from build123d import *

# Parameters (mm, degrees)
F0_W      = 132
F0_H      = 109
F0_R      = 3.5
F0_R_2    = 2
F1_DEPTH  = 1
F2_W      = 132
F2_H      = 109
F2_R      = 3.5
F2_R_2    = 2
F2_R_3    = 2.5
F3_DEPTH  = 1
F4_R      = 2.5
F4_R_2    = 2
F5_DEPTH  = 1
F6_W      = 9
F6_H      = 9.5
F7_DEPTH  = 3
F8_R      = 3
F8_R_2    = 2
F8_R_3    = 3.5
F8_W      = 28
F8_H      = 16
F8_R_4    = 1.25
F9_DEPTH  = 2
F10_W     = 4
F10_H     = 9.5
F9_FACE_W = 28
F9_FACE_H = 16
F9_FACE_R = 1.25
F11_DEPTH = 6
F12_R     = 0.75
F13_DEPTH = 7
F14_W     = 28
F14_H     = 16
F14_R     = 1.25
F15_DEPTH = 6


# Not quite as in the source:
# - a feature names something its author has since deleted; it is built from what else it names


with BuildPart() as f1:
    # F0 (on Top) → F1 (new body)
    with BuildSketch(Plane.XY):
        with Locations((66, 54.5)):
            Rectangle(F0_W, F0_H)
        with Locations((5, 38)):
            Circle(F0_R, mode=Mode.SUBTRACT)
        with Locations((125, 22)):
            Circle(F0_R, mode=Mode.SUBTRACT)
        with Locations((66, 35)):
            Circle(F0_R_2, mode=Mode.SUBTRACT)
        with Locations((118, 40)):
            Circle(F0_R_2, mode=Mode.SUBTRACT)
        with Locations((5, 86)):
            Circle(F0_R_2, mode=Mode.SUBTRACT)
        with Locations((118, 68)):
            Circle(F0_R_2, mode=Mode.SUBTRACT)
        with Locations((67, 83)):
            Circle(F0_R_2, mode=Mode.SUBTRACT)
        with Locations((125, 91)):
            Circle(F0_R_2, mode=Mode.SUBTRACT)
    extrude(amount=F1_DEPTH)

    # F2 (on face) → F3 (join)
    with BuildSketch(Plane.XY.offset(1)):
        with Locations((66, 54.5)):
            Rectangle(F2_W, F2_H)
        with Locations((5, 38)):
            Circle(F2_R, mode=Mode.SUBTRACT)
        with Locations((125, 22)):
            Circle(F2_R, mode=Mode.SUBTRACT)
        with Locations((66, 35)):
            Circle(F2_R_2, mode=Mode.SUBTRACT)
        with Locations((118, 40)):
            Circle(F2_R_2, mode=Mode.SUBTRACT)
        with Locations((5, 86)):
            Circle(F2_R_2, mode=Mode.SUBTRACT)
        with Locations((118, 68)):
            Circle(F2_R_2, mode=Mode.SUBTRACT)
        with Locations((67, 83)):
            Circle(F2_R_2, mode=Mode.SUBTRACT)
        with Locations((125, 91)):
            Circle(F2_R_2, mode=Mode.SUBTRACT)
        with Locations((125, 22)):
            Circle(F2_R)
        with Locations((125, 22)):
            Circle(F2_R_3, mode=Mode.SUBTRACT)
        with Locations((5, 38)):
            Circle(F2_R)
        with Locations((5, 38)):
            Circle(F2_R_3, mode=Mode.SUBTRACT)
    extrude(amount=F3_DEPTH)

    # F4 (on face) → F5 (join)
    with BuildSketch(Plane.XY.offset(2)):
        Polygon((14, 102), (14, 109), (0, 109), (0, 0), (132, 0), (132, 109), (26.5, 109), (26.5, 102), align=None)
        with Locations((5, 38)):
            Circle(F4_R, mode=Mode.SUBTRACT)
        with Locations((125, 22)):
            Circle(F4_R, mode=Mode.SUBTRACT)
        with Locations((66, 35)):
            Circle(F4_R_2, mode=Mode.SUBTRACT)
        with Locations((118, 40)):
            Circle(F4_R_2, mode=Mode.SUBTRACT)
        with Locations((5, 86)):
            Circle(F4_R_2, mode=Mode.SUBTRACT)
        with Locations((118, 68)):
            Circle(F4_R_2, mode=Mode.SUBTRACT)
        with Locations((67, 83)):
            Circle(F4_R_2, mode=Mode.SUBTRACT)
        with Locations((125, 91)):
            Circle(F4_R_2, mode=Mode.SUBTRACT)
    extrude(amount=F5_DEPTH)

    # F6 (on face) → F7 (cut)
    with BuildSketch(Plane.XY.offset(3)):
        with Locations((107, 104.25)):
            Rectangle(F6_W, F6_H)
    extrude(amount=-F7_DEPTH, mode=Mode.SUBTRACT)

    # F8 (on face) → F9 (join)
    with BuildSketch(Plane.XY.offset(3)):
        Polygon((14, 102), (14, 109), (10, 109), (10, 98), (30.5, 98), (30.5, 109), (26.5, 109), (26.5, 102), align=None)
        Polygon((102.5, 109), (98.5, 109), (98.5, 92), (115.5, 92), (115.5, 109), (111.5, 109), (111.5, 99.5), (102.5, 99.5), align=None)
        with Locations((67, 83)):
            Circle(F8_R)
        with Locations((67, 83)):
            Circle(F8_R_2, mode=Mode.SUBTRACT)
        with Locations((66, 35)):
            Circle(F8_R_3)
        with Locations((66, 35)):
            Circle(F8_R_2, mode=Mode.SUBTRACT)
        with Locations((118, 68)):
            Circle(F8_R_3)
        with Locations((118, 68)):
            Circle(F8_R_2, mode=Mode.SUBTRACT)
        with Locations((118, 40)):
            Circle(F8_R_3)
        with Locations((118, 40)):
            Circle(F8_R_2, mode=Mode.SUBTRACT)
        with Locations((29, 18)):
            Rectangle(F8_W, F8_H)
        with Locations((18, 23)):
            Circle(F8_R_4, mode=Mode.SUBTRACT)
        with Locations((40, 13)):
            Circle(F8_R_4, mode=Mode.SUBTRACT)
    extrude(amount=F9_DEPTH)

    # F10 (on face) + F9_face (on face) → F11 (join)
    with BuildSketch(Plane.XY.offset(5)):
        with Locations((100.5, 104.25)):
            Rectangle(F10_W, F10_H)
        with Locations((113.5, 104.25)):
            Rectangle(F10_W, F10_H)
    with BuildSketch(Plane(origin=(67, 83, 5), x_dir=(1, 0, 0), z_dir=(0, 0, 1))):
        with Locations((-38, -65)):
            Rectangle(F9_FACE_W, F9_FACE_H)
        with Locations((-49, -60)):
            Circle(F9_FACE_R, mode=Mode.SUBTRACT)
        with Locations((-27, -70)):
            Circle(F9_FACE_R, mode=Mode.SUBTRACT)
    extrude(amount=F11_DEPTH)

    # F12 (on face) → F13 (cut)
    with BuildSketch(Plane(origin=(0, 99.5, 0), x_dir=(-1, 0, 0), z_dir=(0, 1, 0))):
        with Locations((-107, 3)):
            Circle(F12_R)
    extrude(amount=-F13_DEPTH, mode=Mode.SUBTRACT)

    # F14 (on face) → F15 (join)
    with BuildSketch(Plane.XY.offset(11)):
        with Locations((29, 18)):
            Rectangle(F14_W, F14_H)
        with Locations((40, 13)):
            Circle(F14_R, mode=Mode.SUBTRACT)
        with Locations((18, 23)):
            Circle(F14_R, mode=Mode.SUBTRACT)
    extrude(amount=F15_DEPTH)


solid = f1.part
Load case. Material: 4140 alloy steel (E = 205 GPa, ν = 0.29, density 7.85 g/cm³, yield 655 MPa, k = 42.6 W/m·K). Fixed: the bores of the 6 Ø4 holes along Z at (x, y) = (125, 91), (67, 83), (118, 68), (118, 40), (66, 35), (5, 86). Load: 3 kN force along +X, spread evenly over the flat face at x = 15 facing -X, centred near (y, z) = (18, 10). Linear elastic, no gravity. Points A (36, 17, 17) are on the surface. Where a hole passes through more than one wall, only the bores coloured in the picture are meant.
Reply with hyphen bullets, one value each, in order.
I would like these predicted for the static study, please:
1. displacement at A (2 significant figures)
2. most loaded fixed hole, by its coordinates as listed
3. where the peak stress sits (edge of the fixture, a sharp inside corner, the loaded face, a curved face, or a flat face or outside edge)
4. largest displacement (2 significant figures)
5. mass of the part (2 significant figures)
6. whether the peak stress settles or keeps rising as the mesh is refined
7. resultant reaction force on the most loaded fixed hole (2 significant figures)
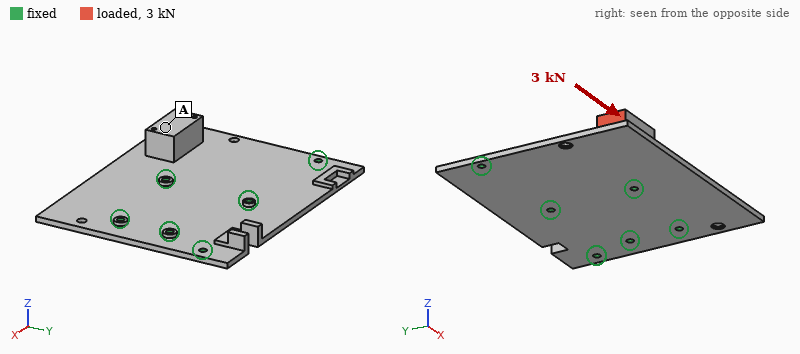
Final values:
- 0.34 mm
- (66, 35)
- edge of the fixture
- 0.84 mm
- 390 g
- keeps rising
- 2.1 kN
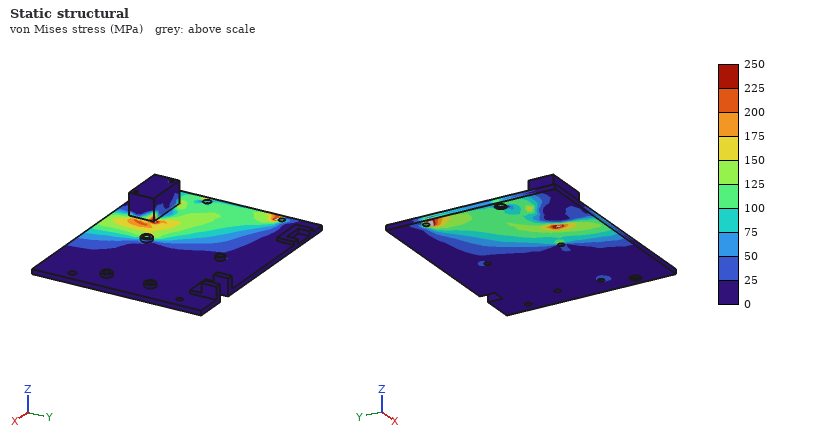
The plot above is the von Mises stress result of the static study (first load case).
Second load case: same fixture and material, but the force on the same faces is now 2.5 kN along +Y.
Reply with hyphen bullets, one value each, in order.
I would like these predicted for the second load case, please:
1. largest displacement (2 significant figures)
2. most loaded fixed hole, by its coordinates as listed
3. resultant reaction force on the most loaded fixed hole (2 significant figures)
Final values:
- 0.61 mm
- (5, 86)
- 1.3 kN
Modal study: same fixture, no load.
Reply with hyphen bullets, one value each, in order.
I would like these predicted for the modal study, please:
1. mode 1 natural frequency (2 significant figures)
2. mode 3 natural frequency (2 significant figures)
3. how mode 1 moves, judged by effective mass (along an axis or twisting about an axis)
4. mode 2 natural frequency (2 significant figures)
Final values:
- 620 Hz
- 2000 Hz
- along Z
- 1600 Hz
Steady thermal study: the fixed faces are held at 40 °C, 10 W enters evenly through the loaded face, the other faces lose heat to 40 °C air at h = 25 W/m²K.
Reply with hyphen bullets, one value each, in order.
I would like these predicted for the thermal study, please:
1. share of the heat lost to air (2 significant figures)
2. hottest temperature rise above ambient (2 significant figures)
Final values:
- 56 %
- 42 K
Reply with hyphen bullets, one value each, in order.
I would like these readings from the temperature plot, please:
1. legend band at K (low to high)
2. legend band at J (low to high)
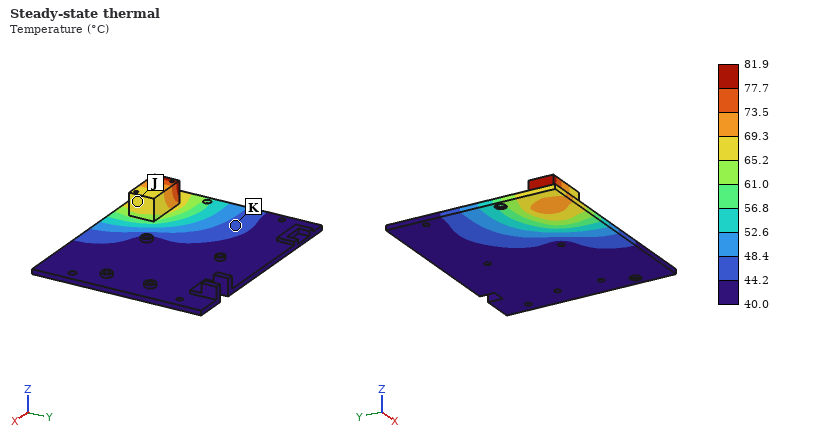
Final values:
- 44.2 to 48.4 °C
- 65.2 to 69.3 °C
